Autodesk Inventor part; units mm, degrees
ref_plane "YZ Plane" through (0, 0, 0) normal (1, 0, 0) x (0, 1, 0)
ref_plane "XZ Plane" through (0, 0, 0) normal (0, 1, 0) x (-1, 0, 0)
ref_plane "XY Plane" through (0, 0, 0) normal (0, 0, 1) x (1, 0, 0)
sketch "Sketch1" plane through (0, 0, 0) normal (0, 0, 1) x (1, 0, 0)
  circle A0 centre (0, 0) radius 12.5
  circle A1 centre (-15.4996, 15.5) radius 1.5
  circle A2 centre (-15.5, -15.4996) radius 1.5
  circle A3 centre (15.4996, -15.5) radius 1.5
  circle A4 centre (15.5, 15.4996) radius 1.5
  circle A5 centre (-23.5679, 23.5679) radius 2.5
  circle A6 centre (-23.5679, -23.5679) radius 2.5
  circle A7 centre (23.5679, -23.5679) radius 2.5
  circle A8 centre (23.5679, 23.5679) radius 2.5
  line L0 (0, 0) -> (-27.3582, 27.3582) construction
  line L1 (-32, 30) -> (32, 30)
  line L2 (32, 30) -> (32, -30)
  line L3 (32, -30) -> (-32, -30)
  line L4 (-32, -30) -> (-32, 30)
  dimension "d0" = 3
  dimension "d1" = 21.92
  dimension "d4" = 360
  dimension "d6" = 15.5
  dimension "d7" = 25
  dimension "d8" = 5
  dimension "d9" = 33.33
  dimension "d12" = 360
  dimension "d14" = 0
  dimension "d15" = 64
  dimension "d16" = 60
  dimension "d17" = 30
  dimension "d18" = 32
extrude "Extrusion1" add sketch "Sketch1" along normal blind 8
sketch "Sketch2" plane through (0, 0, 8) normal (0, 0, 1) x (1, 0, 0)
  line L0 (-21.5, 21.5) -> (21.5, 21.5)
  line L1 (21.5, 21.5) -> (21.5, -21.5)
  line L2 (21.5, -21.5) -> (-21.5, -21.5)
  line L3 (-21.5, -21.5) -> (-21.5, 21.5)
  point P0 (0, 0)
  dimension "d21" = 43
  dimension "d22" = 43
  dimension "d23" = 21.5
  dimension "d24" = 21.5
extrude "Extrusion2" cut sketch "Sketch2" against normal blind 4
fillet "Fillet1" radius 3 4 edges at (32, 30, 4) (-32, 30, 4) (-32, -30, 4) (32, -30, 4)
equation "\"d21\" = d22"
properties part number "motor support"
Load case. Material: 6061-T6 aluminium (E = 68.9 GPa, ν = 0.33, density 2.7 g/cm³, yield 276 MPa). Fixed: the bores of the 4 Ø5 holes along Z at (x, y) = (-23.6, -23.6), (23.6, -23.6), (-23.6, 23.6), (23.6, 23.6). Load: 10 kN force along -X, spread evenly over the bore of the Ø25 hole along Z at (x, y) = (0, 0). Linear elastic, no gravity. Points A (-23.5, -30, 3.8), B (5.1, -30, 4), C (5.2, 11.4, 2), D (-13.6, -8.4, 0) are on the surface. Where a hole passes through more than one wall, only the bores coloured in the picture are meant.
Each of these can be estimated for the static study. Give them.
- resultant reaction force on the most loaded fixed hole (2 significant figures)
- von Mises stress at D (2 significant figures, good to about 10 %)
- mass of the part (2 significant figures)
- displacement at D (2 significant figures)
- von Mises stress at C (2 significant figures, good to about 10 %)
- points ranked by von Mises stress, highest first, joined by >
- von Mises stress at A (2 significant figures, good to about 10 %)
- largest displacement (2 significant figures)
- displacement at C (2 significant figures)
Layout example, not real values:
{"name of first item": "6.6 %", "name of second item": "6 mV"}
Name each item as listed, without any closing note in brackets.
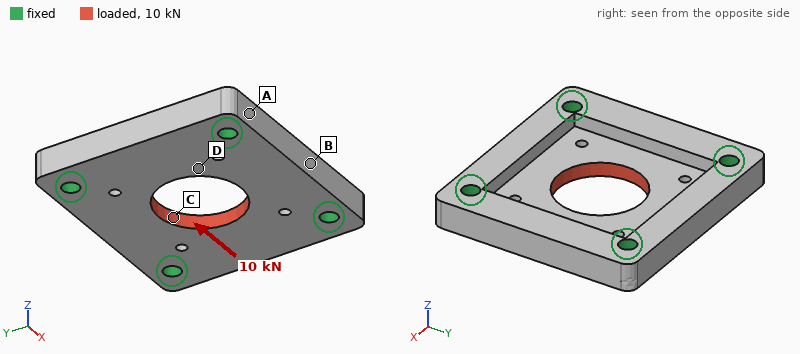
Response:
{"resultant reaction force on the most loaded fixed hole": "2.6 kN", "von Mises stress at D": "34 MPa", "mass of the part": "56 g", "displacement at D": "15 µm", "von Mises stress at C": "57 MPa", "points ranked by von Mises stress, highest first, joined by >": "C > D > A > B", "von Mises stress at A": "17 MPa", "largest displacement": "20 µm", "displacement at C": "14 µm"}
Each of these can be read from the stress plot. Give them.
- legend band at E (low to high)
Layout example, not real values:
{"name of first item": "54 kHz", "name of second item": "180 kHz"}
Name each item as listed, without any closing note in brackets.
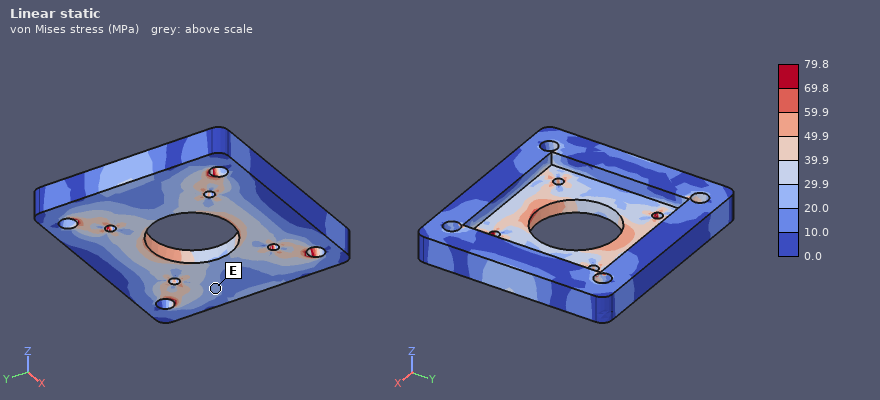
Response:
{"legend band at E": "20.0 to 29.9 MPa"}
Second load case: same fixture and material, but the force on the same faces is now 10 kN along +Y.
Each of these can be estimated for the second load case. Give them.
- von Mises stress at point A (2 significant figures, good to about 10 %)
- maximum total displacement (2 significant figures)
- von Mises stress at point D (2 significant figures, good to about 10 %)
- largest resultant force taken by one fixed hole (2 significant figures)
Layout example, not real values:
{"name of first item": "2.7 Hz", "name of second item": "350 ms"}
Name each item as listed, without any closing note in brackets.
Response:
{"von Mises stress at point A": "28 MPa", "maximum total displacement": "21 µm", "von Mises stress at point D": "36 MPa", "largest resultant force taken by one fixed hole": "2.7 kN"}
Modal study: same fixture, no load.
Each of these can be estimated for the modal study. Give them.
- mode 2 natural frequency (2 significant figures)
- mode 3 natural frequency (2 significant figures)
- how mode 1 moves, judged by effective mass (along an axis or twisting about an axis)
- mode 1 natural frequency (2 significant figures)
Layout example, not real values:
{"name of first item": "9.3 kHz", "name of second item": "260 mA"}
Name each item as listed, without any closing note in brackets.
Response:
{"mode 2 natural frequency": "15 kHz", "mode 3 natural frequency": "15 kHz", "how mode 1 moves, judged by effective mass": "along Z", "mode 1 natural frequency": "13 kHz"}
